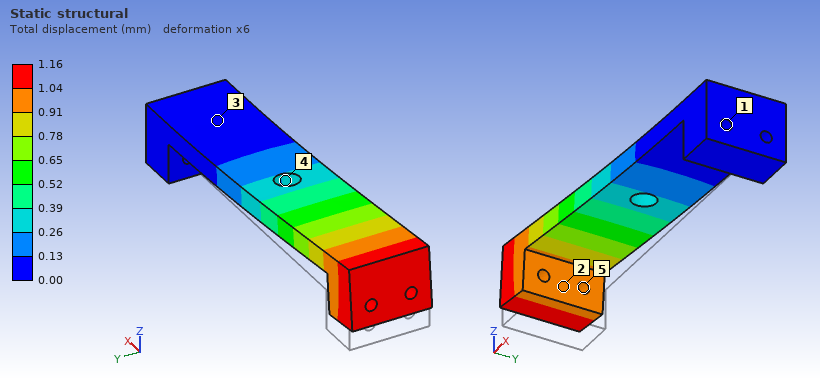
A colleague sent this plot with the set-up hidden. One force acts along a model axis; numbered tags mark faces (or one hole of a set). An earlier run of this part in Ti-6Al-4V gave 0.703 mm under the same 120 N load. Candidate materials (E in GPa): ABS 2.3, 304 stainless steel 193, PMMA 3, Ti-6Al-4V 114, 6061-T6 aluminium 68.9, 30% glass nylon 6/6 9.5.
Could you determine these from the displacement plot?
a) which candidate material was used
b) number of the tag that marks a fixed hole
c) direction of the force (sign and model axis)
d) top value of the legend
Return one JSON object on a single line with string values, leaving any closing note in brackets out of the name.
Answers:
{"which candidate material was used": "6061-T6 aluminium", "number of the tag that marks a fixed hole": "1", "direction of the force": "+Z", "top value of the legend": "1.16 mm"}
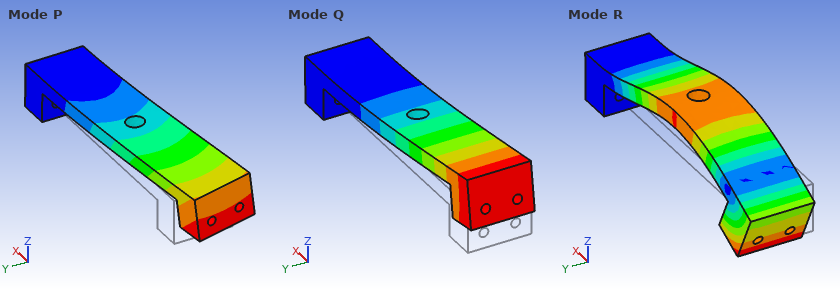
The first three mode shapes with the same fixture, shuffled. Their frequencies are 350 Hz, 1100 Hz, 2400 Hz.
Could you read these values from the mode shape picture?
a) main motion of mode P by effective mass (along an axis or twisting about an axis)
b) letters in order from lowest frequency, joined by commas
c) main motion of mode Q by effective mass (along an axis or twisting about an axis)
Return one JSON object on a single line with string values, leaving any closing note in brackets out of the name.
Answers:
{"main motion of mode P by effective mass": "along Y", "letters in order from lowest frequency, joined by commas": "Q, P, R", "main motion of mode Q by effective mass": "along Z"}
